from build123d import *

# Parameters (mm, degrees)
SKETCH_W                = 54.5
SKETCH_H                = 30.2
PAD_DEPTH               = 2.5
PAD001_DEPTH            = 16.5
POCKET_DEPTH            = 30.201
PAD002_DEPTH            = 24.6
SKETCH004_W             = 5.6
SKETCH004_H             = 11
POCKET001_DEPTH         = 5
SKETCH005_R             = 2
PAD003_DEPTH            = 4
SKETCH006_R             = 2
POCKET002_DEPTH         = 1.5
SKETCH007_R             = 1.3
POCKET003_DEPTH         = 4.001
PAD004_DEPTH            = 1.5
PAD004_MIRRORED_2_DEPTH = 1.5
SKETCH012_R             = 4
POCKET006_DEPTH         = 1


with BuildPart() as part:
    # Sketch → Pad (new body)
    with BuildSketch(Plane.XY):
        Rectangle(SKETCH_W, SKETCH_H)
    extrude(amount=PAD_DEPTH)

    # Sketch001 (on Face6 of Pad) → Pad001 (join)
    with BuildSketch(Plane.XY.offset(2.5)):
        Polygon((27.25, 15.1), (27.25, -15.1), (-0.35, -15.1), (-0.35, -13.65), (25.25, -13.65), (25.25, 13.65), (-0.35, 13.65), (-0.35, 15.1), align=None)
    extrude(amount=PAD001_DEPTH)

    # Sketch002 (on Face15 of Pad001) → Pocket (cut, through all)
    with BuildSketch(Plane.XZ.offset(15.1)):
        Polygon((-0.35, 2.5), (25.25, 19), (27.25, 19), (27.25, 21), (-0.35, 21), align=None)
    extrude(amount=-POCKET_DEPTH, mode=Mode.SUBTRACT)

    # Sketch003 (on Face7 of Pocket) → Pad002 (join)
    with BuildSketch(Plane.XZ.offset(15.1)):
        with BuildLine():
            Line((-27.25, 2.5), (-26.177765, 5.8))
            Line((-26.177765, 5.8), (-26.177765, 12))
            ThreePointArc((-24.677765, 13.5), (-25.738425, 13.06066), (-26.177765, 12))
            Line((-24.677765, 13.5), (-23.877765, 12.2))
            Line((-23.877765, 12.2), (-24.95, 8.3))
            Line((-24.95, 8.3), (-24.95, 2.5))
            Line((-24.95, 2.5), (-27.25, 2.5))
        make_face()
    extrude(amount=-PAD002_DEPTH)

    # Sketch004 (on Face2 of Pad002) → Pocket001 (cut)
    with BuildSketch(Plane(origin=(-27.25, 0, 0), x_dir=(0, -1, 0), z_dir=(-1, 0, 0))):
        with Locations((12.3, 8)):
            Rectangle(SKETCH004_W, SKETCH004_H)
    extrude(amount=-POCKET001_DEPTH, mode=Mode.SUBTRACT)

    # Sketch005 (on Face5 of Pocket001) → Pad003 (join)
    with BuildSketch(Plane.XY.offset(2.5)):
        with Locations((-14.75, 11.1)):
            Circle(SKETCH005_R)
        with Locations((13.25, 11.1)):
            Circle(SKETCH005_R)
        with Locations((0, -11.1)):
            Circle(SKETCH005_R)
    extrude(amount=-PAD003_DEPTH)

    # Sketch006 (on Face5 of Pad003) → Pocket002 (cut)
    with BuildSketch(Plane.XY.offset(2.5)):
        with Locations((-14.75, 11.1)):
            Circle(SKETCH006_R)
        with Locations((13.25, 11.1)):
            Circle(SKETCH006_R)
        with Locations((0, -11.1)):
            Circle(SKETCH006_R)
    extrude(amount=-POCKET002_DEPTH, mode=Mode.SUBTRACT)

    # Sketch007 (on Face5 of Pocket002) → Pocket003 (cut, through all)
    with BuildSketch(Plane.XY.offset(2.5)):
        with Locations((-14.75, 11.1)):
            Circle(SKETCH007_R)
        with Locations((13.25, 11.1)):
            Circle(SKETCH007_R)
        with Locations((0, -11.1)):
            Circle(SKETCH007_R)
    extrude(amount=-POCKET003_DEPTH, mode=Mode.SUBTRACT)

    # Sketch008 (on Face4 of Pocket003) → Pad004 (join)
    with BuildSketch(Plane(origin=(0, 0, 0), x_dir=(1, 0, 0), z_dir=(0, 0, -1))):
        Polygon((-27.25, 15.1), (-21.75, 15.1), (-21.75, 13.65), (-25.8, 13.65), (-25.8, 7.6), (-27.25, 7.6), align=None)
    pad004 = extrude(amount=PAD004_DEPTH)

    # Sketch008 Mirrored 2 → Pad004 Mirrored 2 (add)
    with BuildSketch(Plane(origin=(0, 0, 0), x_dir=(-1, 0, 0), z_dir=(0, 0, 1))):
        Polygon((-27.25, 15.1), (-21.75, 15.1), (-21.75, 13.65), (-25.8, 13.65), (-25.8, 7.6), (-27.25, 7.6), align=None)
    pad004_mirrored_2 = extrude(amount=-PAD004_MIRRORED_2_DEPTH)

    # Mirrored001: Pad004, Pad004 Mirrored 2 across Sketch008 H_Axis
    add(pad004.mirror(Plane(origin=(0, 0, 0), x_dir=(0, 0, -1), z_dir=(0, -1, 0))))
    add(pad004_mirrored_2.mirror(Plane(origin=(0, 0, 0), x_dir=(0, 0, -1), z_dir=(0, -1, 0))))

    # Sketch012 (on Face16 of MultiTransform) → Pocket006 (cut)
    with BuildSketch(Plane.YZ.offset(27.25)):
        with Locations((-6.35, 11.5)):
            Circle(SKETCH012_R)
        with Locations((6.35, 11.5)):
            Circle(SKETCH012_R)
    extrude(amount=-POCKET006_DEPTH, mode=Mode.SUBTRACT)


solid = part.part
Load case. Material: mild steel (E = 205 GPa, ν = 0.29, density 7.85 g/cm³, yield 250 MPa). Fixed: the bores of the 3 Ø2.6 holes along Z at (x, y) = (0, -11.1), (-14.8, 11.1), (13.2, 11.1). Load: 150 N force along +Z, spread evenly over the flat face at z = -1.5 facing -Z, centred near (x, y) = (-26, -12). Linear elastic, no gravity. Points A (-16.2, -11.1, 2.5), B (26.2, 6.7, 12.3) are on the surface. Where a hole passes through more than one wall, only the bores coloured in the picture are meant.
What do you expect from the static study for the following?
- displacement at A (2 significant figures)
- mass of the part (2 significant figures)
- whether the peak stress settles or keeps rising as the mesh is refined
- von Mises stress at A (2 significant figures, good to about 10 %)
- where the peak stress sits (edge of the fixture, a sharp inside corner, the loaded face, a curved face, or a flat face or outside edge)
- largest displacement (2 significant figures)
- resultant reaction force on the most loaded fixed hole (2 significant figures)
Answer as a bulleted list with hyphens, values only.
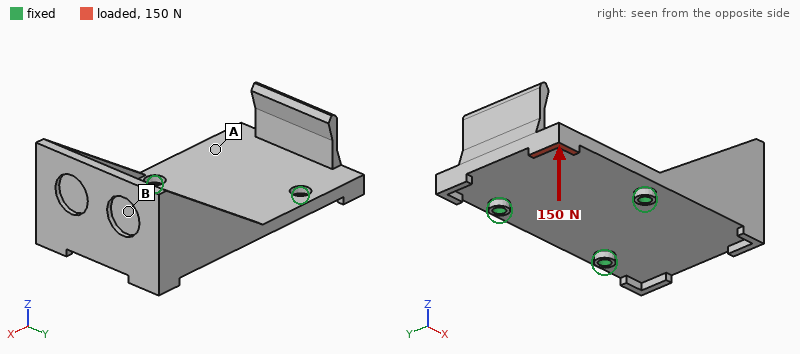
- 0.048 mm
- 47 g
- keeps rising
- 66 MPa
- a sharp inside corner
- 0.12 mm
- 240 N
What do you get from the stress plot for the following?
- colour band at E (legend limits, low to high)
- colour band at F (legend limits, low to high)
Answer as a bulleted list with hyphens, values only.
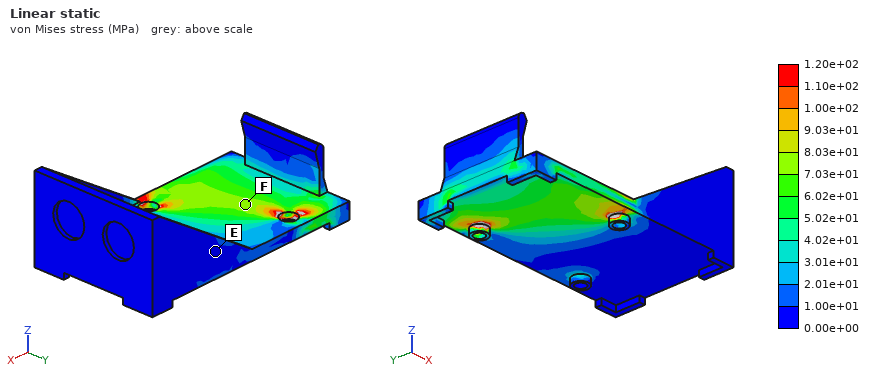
- 0.00e+00 to 1.00e+01 MPa
- 7.03e+01 to 8.03e+01 MPa
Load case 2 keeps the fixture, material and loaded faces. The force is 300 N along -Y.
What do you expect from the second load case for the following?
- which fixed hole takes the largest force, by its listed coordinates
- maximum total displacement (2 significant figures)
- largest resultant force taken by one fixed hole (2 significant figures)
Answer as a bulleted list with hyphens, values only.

- (-14.8, 11.1)
- 26 µm
- 320 N
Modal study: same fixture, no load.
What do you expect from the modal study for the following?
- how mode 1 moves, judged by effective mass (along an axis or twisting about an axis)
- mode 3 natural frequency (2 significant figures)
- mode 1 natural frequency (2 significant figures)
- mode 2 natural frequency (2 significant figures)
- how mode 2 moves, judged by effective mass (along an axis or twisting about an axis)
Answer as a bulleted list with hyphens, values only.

- along Z
- 6000 Hz
- 2500 Hz
- 3300 Hz
- along Z
